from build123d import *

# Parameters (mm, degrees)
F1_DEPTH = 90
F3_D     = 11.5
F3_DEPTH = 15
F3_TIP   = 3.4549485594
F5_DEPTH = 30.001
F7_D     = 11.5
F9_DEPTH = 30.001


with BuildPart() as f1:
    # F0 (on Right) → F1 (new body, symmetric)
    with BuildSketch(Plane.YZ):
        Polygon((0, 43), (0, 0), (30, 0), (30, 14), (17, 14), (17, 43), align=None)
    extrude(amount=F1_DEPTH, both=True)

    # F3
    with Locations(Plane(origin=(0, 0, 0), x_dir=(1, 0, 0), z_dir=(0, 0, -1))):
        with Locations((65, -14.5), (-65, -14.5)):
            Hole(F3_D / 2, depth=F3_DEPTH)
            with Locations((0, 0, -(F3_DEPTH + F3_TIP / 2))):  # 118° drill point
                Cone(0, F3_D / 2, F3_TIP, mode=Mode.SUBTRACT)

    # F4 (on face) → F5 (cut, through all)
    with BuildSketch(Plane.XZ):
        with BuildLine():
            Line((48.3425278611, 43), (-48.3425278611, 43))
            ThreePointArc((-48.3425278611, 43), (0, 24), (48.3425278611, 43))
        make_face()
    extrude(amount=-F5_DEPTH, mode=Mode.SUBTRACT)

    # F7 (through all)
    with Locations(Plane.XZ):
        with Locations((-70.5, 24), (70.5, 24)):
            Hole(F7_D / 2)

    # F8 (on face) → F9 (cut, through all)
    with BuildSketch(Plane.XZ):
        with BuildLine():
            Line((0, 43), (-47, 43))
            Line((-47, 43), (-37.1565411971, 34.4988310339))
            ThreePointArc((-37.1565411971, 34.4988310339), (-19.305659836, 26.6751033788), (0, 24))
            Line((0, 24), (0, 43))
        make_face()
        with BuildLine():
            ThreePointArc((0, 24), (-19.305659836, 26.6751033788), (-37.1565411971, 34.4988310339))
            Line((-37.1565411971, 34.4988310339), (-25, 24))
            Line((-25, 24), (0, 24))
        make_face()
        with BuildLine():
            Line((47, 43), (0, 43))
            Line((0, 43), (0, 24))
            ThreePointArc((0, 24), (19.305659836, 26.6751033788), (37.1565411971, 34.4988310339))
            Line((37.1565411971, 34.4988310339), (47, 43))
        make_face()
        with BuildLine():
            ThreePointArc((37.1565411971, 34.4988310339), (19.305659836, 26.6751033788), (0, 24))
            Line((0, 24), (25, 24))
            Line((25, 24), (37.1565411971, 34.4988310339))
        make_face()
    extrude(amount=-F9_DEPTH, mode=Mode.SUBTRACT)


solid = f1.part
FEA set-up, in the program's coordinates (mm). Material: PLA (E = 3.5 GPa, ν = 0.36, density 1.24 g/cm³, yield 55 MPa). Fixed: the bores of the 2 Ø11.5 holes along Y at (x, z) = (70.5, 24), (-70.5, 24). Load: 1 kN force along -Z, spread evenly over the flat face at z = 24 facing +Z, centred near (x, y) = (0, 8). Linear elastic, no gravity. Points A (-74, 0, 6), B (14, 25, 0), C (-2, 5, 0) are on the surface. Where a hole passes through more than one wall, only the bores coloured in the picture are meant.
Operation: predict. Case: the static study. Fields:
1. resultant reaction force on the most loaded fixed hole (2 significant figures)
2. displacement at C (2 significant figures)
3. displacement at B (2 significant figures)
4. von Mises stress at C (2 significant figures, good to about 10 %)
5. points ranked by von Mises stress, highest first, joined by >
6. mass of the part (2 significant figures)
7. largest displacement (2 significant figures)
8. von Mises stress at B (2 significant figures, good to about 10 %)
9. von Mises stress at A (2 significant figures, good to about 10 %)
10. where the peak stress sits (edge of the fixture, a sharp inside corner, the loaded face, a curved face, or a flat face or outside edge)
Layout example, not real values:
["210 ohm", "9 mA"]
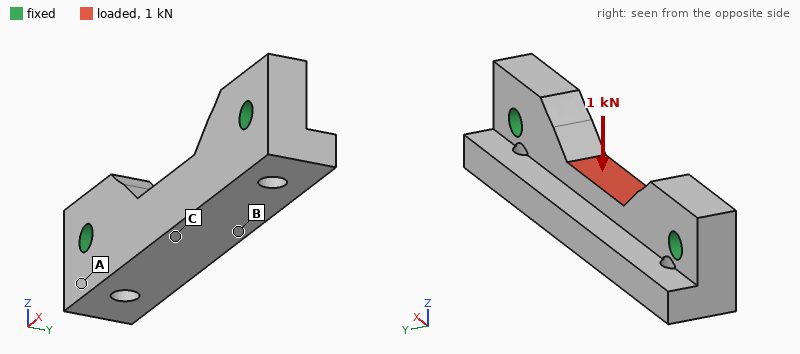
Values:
["790 N", "0.13 mm", "0.12 mm", "5.6 MPa", "C > B > A", "170 g", "0.15 mm", "2.9 MPa", "1.2 MPa", "edge of the fixture"]
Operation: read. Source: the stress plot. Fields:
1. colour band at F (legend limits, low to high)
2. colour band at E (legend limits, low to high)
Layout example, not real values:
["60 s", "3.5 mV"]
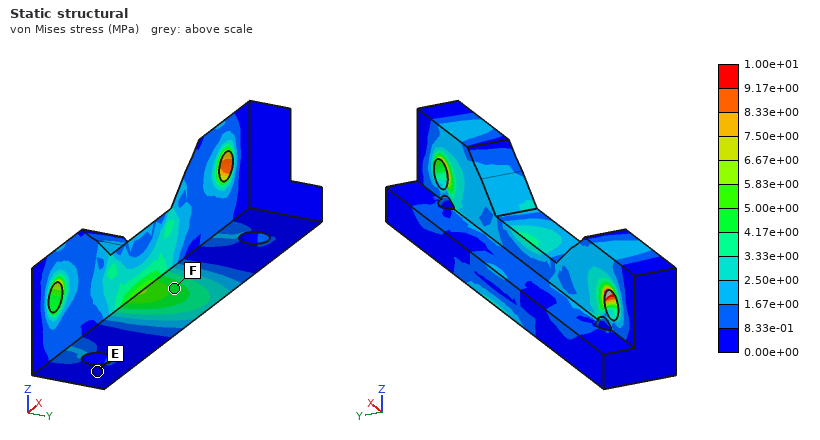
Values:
["4.17e+00 to 5.00e+00 MPa", "0.00e+00 to 8.33e-01 MPa"]
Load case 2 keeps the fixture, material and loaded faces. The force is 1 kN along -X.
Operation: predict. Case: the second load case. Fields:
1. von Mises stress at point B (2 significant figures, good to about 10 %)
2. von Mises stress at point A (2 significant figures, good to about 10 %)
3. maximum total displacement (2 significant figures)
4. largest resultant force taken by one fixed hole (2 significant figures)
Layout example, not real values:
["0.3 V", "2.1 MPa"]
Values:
["0.69 MPa", "0.51 MPa", "36 µm", "500 N"]
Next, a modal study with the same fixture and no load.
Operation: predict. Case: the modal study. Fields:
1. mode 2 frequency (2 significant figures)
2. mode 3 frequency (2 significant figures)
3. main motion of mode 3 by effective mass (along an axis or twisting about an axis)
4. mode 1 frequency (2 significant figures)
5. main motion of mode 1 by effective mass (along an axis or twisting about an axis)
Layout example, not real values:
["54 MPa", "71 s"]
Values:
["2000 Hz", "2900 Hz", "twisting about X", "1500 Hz", "along Y"]
